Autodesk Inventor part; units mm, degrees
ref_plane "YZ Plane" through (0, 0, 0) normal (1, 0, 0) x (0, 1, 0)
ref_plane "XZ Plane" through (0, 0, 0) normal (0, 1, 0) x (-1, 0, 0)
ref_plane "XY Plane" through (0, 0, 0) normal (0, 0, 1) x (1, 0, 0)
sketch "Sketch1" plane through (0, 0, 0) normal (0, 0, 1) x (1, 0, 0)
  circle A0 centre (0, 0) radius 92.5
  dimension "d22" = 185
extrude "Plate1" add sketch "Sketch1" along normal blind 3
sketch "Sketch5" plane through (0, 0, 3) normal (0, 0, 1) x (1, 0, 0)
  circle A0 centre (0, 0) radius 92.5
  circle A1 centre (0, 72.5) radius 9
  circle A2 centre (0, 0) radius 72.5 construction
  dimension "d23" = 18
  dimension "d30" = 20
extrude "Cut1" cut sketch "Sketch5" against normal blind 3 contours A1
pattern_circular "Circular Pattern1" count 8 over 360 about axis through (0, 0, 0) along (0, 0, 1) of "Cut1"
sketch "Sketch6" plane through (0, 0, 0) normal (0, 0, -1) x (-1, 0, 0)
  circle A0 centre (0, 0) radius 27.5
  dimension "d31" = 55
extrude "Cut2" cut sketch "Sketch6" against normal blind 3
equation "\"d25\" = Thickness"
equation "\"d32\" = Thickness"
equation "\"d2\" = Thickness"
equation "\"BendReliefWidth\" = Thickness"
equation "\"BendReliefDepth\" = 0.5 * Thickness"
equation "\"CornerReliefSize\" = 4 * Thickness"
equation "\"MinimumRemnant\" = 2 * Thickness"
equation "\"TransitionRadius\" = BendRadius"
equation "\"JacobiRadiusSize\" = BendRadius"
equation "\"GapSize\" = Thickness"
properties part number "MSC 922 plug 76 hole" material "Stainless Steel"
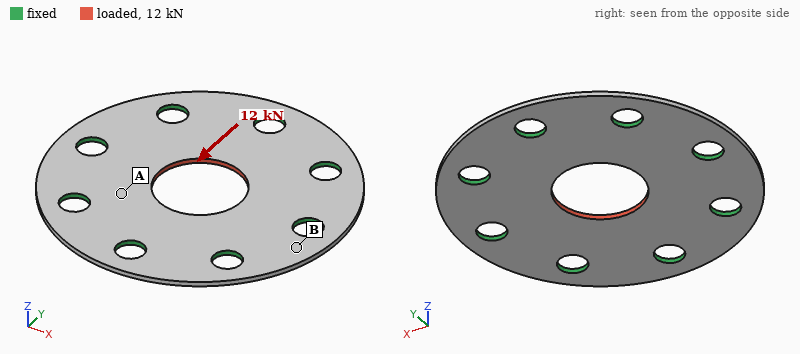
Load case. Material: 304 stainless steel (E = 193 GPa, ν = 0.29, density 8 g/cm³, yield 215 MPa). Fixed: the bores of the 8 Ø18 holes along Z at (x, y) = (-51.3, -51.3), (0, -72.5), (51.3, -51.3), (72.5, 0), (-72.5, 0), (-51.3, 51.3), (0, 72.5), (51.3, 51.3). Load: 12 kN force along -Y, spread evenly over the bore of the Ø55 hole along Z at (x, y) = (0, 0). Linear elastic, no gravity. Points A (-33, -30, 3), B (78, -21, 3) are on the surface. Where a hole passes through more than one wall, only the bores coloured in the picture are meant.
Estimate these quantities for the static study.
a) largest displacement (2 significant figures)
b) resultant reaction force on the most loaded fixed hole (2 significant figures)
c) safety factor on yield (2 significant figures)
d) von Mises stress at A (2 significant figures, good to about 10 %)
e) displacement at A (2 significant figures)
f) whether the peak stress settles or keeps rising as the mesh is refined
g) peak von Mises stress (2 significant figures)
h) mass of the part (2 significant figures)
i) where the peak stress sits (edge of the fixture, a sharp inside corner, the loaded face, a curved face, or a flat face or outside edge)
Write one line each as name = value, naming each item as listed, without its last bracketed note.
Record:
largest displacement = 5.1 µm
resultant reaction force on the most loaded fixed hole = 2.4 kN
safety factor on yield = 5.4
von Mises stress at A = 19 MPa
displacement at A = 2.2 µm
whether the peak stress settles or keeps rising as the mesh is refined = settles
peak von Mises stress = 40 MPa
mass of the part = 540 g
where the peak stress sits = the loaded face
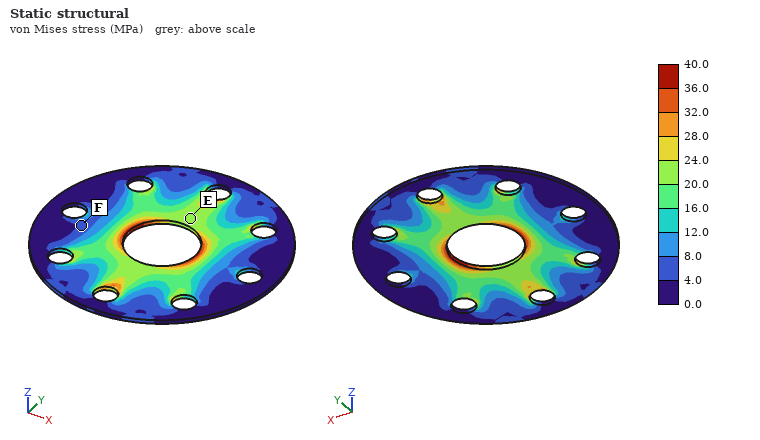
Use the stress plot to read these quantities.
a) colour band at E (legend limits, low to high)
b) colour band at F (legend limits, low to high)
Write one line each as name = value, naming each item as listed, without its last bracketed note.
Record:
colour band at E = 20.0 to 24.0 MPa
colour band at F = 4.0 to 8.0 MPa
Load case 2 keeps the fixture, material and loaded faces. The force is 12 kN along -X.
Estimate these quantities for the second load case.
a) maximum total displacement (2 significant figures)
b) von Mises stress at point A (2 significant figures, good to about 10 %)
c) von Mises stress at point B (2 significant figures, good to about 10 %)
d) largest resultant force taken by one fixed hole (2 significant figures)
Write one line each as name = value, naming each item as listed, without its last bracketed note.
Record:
maximum total displacement = 5.1 µm
von Mises stress at point A = 18 MPa
von Mises stress at point B = 6.2 MPa
largest resultant force taken by one fixed hole = 2.4 kN
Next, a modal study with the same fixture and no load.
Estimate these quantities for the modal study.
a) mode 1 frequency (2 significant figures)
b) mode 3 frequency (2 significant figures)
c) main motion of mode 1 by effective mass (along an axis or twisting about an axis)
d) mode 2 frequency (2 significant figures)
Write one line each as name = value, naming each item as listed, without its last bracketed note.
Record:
mode 1 frequency = 2200 Hz
mode 3 frequency = 3000 Hz
main motion of mode 1 by effective mass = along Z
mode 2 frequency = 3000 Hz
